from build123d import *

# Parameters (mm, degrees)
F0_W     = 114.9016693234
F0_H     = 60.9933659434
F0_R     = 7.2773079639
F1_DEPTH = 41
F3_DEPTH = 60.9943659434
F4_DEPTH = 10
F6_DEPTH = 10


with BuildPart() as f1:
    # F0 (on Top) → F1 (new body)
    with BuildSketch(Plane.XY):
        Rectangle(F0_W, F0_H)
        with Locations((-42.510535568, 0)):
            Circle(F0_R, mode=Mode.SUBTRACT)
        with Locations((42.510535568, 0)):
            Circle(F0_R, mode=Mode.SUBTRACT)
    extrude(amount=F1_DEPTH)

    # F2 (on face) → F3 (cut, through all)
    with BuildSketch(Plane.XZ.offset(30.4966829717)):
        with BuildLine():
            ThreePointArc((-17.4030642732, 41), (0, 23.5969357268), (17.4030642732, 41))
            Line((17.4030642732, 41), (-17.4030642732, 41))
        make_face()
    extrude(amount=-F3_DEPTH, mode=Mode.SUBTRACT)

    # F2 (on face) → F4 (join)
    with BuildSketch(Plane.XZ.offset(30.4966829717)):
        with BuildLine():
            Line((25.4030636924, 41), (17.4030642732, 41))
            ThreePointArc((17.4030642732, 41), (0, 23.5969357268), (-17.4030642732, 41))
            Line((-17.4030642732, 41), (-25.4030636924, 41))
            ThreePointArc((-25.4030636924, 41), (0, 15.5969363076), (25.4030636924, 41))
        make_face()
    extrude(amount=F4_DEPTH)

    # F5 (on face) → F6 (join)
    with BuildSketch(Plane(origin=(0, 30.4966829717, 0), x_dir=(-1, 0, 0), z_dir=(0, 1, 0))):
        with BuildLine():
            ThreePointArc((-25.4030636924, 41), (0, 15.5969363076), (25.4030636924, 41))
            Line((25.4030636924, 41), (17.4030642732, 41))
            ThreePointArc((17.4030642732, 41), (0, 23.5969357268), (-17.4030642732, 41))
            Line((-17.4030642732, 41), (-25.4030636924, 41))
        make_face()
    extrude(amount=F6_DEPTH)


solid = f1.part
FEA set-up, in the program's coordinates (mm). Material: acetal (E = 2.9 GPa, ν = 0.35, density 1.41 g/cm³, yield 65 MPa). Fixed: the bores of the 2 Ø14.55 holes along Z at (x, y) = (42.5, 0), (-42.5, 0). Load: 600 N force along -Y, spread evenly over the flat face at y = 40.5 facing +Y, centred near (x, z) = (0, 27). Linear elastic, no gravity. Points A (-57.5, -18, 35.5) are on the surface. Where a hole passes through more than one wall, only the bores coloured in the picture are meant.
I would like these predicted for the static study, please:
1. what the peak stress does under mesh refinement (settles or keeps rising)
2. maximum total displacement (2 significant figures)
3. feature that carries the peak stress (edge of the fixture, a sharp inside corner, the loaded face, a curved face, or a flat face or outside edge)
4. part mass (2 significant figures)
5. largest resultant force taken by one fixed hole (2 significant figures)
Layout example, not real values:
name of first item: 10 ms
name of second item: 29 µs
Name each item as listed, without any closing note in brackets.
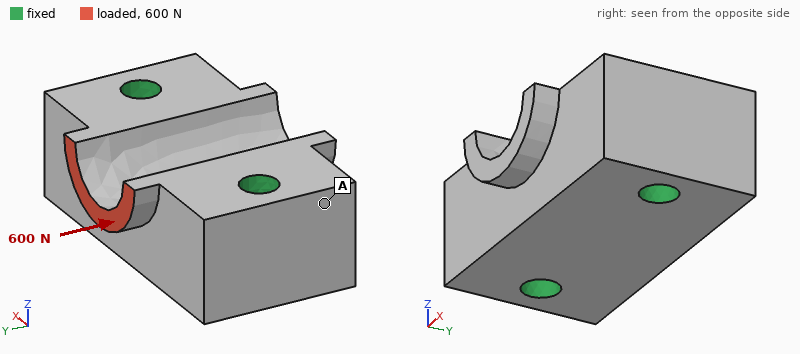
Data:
what the peak stress does under mesh refinement: keeps rising
maximum total displacement: 20 µm
feature that carries the peak stress: a sharp inside corner
part mass: 360 g
largest resultant force taken by one fixed hole: 310 N
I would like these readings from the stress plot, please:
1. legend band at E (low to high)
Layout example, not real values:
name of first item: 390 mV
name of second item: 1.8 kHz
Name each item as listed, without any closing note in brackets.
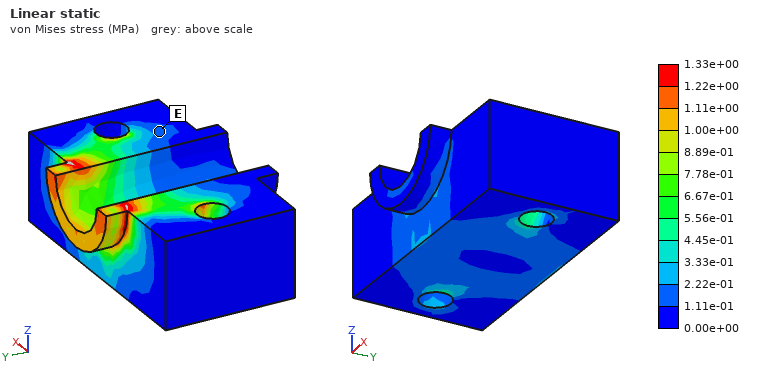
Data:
legend band at E: 1.11e-01 to 2.22e-01 MPa
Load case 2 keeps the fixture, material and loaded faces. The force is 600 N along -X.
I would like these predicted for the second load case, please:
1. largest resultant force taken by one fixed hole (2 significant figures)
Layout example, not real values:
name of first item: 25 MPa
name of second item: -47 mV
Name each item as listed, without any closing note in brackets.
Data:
largest resultant force taken by one fixed hole: 390 N
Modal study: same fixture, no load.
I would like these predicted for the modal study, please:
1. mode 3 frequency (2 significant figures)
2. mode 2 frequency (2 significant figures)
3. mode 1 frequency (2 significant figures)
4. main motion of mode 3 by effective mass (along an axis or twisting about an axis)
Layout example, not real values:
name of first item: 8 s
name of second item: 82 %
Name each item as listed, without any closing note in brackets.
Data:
mode 3 frequency: 4300 Hz
mode 2 frequency: 3800 Hz
mode 1 frequency: 3700 Hz
main motion of mode 3 by effective mass: along Y
